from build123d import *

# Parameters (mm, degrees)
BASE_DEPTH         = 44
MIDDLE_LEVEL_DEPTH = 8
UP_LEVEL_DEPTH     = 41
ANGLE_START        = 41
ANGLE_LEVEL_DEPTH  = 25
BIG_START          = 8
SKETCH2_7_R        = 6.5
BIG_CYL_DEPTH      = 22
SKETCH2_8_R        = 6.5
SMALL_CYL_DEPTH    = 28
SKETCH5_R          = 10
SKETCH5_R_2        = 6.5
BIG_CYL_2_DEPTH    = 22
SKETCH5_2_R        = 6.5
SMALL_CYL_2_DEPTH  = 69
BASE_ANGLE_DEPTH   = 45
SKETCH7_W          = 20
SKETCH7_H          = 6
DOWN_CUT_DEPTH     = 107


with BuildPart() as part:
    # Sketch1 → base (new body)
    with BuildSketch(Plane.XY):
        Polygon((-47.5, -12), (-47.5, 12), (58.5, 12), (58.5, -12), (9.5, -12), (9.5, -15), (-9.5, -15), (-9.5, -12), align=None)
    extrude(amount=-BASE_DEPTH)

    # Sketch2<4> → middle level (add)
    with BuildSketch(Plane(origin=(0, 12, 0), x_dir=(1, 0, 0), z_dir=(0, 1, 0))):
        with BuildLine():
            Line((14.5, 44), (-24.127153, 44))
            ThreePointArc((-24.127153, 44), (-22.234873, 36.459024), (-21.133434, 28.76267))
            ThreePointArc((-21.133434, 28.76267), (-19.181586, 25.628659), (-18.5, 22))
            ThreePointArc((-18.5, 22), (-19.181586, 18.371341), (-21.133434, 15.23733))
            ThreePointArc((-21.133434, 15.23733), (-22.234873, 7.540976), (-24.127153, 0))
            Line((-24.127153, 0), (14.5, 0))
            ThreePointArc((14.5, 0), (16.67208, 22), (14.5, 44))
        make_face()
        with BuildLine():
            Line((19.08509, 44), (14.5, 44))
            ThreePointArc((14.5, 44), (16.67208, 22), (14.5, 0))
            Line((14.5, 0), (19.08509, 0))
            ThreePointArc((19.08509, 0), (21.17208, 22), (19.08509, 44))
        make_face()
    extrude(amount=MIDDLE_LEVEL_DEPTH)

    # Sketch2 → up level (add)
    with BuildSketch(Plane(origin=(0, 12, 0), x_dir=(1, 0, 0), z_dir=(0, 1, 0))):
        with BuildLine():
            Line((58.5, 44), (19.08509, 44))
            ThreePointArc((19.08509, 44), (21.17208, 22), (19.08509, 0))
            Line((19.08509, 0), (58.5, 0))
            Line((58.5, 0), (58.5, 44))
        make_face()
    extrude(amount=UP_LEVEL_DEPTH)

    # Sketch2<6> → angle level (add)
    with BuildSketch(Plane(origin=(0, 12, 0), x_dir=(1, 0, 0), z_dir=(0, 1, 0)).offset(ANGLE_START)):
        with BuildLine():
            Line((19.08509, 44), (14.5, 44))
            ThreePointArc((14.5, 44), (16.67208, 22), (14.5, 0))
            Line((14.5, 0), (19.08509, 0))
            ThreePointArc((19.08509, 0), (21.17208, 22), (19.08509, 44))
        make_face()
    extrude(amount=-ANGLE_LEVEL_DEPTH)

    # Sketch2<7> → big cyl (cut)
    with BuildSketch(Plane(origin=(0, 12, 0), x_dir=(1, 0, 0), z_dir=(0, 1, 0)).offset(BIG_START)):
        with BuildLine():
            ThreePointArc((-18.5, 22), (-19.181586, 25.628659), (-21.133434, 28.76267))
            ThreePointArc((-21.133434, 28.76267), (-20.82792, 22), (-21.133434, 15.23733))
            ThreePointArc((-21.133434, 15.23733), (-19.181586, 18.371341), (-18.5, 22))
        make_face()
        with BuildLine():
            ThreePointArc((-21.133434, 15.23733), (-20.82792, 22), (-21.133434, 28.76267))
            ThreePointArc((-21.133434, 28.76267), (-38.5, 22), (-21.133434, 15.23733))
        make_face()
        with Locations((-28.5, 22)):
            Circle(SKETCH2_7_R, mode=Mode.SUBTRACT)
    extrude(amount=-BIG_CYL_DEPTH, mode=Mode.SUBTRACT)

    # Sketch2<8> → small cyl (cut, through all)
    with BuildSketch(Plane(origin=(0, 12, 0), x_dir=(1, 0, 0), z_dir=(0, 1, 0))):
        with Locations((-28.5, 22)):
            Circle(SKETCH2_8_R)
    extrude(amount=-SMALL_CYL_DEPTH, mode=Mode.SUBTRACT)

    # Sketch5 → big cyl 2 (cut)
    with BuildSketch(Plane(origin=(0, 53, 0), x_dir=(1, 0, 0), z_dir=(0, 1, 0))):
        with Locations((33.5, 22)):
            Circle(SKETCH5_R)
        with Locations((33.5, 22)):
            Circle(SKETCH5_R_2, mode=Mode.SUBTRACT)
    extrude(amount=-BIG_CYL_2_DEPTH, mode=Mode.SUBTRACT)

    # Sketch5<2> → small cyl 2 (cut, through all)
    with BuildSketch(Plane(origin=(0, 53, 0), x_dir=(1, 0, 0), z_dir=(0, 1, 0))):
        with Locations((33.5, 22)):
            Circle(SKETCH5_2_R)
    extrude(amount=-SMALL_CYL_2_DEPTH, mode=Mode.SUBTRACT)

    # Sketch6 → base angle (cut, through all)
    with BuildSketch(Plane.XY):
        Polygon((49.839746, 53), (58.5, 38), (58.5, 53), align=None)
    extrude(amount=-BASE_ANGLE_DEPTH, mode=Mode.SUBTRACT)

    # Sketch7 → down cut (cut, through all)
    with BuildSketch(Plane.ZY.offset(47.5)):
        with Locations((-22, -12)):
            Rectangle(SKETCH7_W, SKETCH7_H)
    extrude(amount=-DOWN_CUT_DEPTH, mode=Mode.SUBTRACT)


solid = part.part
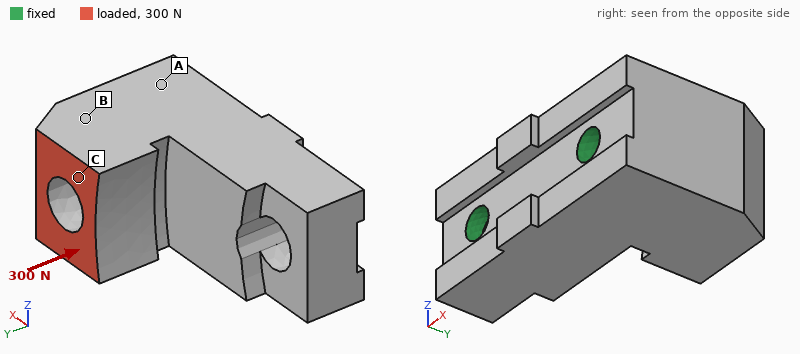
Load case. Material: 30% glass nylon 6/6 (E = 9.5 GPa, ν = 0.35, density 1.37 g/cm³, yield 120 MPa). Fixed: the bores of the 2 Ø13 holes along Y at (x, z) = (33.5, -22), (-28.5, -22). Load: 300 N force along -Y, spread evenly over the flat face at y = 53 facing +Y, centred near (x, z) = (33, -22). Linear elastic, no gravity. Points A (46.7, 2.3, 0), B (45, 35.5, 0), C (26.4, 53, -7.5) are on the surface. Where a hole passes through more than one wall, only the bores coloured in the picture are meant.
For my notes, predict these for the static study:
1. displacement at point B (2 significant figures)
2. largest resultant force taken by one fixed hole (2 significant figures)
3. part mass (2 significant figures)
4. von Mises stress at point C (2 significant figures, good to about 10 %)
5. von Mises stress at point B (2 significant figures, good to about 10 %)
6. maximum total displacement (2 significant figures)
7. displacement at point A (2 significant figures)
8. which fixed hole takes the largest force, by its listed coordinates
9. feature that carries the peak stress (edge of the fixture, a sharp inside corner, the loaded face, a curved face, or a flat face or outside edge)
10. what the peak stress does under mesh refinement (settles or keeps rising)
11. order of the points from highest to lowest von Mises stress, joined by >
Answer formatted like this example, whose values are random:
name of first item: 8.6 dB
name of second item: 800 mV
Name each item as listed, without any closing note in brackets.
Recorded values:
displacement at point B: 0.63 µm
largest resultant force taken by one fixed hole: 290 N
part mass: 240 g
von Mises stress at point C: 0.27 MPa
von Mises stress at point B: 0.16 MPa
maximum total displacement: 1.9 µm
displacement at point A: 0.30 µm
which fixed hole takes the largest force, by its listed coordinates: (33.5, -22)
feature that carries the peak stress: edge of the fixture
what the peak stress does under mesh refinement: keeps rising
order of the points from highest to lowest von Mises stress, joined by >: C > B > A
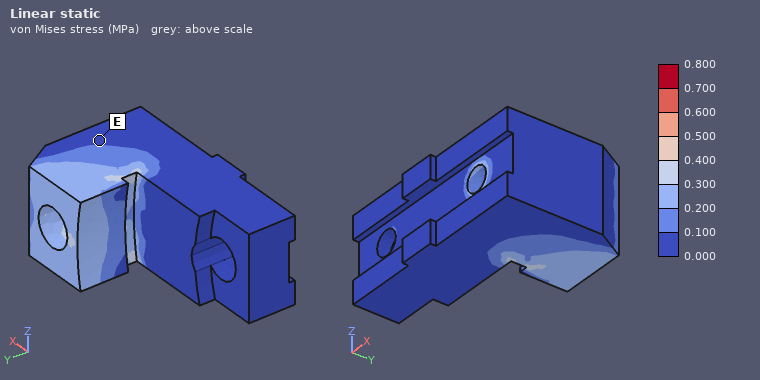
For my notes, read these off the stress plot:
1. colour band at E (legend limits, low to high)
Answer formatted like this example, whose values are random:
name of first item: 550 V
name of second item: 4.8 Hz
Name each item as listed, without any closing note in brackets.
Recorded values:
colour band at E: 0.000 to 0.100 MPa
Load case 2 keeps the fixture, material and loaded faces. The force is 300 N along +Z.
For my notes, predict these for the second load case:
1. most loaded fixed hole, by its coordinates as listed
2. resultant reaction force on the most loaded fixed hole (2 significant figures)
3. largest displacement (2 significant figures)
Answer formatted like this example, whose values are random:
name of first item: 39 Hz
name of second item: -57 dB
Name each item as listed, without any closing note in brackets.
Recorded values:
most loaded fixed hole, by its coordinates as listed: (33.5, -22)
resultant reaction force on the most loaded fixed hole: 310 N
largest displacement: 8.7 µm
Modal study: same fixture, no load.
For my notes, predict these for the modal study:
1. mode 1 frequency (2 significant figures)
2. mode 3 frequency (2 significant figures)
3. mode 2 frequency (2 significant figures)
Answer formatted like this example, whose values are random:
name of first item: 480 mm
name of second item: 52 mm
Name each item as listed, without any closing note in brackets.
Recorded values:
mode 1 frequency: 5300 Hz
mode 3 frequency: 6800 Hz
mode 2 frequency: 6500 Hz
